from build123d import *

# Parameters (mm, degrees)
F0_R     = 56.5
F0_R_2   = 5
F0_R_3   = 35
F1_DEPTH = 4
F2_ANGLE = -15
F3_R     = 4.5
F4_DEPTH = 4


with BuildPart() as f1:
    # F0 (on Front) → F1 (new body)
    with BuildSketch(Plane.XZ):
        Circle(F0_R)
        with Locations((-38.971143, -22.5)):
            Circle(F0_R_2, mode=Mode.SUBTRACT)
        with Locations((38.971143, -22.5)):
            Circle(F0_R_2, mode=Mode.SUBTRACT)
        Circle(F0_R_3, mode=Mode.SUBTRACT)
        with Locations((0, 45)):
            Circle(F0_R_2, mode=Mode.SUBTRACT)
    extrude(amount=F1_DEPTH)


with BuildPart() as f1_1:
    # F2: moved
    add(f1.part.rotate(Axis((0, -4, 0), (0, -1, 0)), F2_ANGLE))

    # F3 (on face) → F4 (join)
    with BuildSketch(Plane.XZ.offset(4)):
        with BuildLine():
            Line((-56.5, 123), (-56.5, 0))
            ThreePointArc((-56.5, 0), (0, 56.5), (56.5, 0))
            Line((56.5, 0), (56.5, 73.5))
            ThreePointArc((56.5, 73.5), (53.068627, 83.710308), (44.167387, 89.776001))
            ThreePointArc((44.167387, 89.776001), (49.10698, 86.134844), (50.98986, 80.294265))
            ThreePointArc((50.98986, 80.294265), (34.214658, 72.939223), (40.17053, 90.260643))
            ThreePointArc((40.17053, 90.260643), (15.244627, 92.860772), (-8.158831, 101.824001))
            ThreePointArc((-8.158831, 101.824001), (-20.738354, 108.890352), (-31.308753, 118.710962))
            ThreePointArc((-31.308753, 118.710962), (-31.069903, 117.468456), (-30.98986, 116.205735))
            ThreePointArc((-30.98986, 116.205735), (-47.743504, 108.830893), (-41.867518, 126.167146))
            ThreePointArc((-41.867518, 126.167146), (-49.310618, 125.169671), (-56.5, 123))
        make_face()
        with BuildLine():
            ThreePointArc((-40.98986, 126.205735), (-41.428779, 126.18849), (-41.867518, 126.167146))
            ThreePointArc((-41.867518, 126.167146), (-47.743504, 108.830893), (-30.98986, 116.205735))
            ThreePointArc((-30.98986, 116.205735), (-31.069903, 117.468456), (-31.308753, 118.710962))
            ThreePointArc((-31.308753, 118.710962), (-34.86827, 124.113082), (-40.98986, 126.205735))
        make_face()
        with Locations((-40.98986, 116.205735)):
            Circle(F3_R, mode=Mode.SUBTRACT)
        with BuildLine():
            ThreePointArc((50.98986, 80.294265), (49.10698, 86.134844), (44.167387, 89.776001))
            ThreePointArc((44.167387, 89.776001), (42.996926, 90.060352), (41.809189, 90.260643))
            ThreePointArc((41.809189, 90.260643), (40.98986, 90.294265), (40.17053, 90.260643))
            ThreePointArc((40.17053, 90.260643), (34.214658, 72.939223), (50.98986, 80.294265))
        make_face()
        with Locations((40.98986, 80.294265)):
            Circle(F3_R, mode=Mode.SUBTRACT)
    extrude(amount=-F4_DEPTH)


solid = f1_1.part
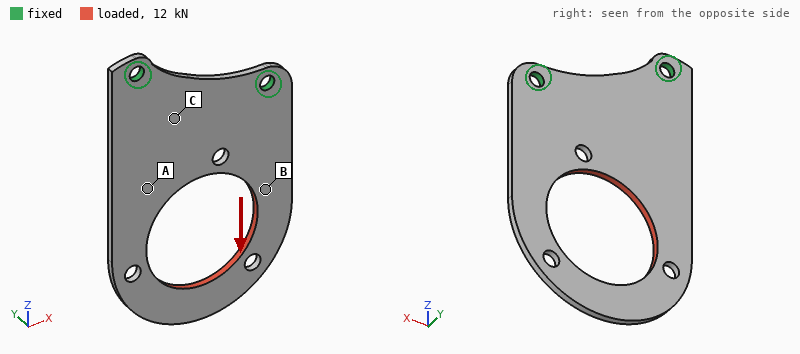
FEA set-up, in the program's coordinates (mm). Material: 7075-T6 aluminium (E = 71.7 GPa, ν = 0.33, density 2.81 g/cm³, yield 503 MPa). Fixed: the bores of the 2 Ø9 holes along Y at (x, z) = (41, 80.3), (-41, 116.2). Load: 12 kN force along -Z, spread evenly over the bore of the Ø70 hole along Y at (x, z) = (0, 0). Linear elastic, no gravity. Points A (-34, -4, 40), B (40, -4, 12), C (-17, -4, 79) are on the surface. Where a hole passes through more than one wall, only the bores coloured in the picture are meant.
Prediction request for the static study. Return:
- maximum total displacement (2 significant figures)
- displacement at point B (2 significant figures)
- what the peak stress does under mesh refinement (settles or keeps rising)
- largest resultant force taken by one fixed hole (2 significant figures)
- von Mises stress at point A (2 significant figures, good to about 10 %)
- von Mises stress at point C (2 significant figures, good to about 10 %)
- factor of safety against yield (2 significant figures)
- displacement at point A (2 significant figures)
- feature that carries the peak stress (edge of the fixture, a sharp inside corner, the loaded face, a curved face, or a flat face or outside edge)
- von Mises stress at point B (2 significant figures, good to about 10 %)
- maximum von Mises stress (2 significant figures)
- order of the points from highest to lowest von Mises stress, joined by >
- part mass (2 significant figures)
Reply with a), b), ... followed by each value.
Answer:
a) 0.14 mm
b) 0.046 mm
c) settles
d) 6.2 kN
e) 35 MPa
f) 15 MPa
g) 2.9
h) 0.046 mm
i) a curved face
j) 54 MPa
k) 170 MPa
l) B > A > C
m) 140 g
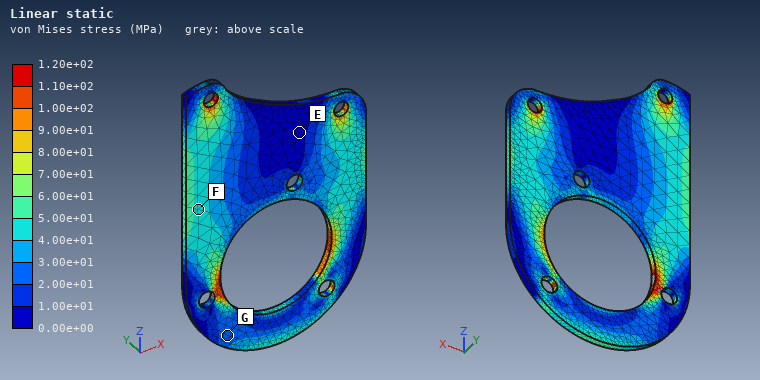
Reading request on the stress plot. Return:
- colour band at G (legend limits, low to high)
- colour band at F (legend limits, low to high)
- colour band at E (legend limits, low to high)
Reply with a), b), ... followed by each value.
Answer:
a) 2.00e+01 to 3.00e+01 MPa
b) 4.00e+01 to 5.00e+01 MPa
c) 0.00e+00 to 1.00e+01 MPa
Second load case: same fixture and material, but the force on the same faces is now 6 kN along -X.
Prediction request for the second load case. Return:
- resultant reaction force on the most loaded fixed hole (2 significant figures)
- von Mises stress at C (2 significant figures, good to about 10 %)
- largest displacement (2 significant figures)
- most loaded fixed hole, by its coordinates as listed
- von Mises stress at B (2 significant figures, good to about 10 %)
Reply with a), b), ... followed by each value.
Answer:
a) 7.7 kN
b) 21 MPa
c) 0.38 mm
d) (41, 80.3)
e) 44 MPa
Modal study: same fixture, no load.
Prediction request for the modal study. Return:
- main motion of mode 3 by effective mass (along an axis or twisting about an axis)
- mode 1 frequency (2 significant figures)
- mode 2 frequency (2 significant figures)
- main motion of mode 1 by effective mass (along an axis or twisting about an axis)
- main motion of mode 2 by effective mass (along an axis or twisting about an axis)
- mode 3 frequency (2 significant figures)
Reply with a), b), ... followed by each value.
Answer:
a) along Y
b) 190 Hz
c) 470 Hz
d) along Y
e) twisting about Z
f) 820 Hz
